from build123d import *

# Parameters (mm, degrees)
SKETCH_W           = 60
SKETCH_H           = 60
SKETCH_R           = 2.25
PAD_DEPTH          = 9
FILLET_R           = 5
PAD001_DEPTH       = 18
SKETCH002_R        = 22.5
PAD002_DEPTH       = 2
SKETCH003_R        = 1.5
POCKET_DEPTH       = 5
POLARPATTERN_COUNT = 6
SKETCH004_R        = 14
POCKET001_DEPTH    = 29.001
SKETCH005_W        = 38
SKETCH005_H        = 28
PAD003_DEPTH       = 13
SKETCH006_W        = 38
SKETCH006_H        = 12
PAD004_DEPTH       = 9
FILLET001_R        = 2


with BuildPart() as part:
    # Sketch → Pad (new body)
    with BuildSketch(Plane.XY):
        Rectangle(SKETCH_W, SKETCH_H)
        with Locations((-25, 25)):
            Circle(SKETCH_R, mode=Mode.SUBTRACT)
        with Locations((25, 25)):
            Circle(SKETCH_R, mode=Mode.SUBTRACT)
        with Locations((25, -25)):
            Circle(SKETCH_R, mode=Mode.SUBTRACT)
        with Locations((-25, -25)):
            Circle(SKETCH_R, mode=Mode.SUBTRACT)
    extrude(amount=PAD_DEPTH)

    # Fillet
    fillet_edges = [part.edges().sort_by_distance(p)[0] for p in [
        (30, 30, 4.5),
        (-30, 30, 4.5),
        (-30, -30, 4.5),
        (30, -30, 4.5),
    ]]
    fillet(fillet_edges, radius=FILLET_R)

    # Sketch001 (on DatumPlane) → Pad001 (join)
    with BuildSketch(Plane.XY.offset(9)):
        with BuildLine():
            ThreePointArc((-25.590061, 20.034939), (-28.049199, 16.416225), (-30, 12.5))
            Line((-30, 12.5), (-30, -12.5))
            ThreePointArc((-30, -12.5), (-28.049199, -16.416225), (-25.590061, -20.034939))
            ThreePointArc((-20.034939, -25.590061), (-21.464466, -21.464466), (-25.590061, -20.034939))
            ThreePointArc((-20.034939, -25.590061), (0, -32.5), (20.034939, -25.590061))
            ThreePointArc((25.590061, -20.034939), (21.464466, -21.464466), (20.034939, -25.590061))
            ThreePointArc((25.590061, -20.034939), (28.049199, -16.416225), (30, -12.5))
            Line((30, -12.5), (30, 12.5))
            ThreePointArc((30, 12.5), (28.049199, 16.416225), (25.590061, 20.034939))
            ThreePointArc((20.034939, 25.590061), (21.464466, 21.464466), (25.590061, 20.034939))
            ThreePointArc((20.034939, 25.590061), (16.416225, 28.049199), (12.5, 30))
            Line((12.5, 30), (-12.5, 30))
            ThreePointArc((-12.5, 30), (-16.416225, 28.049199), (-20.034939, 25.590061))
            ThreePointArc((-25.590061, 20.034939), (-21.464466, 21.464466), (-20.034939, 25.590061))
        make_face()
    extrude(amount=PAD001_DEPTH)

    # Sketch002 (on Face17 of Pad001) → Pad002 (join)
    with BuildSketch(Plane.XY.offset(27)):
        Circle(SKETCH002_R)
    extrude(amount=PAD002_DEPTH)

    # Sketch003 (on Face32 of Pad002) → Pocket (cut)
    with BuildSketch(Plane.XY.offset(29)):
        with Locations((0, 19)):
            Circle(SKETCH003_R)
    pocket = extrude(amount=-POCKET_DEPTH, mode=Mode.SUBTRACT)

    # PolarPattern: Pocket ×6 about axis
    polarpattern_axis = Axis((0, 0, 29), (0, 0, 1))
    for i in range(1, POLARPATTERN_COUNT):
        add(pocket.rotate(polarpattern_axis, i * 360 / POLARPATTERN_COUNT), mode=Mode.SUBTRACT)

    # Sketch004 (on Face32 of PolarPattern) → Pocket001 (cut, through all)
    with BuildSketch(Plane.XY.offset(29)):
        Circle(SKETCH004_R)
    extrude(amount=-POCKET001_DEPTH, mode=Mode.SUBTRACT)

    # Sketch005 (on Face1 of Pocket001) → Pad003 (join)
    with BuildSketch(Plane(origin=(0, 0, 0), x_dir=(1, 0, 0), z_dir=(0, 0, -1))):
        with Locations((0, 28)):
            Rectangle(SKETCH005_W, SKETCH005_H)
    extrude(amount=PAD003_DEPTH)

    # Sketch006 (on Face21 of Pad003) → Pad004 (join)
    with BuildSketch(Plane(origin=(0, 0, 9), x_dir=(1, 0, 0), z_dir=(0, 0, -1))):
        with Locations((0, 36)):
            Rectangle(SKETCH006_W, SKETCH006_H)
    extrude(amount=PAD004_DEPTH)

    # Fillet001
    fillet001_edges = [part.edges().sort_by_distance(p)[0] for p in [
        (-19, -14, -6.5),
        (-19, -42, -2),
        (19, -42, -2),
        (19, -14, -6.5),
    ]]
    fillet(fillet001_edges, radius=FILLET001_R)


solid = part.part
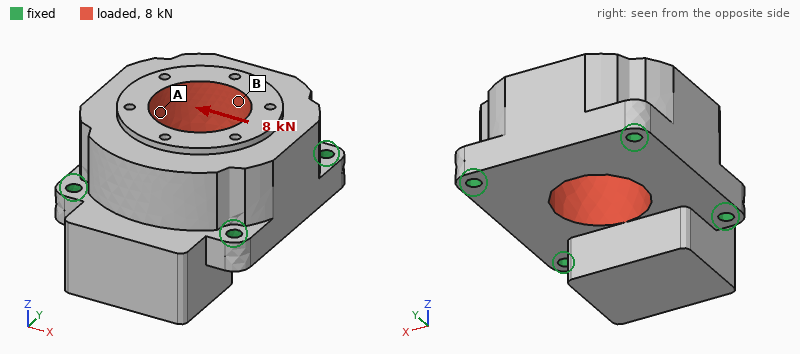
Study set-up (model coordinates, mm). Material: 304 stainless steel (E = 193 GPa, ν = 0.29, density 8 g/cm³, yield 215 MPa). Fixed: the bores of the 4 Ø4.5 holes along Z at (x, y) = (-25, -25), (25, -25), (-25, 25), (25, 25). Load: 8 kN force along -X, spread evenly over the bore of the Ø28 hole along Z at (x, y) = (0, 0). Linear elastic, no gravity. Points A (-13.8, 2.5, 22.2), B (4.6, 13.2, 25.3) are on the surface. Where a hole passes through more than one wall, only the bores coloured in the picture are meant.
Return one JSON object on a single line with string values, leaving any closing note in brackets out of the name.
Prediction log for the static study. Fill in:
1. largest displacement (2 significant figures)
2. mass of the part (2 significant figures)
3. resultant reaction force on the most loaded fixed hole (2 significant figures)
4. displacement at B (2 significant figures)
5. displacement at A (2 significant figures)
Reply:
{"largest displacement": "2.9 µm", "mass of the part": "730 g", "resultant reaction force on the most loaded fixed hole": "2.3 kN", "displacement at B": "2.3 µm", "displacement at A": "2.5 µm"}
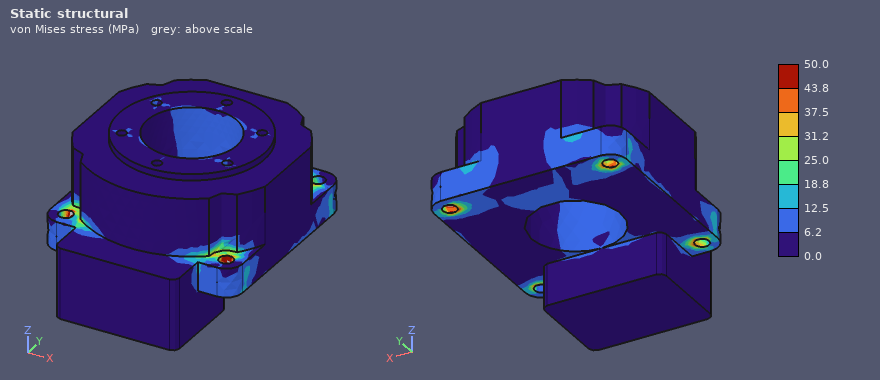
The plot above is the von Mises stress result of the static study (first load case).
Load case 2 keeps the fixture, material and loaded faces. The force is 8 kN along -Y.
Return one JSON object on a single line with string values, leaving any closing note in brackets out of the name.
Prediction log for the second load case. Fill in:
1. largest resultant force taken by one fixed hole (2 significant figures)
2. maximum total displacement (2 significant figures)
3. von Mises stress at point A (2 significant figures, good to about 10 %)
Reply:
{"largest resultant force taken by one fixed hole": "2.3 kN", "maximum total displacement": "2.9 µm", "von Mises stress at point A": "8.5 MPa"}
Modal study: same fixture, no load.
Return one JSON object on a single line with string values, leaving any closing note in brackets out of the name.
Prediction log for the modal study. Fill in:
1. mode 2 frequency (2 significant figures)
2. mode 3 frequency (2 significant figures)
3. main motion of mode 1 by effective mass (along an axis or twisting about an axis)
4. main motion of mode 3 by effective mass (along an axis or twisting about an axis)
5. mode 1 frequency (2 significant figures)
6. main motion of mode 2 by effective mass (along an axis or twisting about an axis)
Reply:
{"mode 2 frequency": "12 kHz", "mode 3 frequency": "13 kHz", "main motion of mode 1 by effective mass": "along Z", "main motion of mode 3 by effective mass": "along X", "mode 1 frequency": "9900 Hz", "main motion of mode 2 by effective mass": "along Z"}
